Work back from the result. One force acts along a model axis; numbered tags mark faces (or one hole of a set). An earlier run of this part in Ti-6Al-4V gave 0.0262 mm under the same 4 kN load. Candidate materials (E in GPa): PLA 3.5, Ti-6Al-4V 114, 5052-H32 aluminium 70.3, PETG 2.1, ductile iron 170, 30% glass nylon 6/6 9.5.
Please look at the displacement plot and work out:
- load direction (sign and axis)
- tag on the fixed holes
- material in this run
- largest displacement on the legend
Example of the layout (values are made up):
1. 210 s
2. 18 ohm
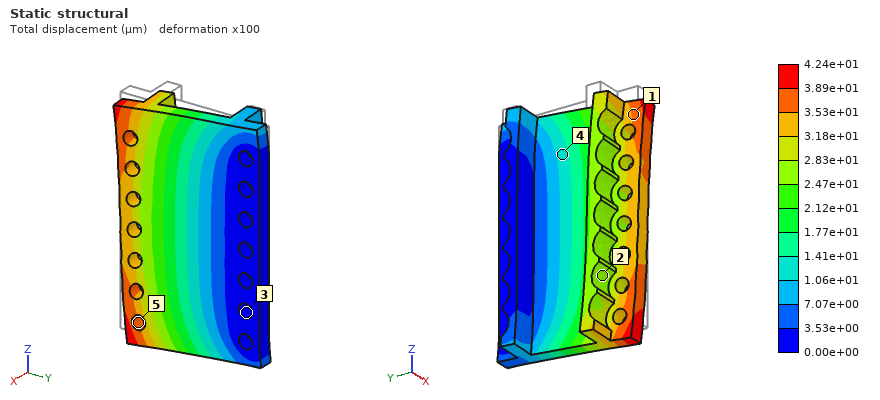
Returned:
1. -Z
2. 3
3. 5052-H32 aluminium
4. 4.24e+01 µm
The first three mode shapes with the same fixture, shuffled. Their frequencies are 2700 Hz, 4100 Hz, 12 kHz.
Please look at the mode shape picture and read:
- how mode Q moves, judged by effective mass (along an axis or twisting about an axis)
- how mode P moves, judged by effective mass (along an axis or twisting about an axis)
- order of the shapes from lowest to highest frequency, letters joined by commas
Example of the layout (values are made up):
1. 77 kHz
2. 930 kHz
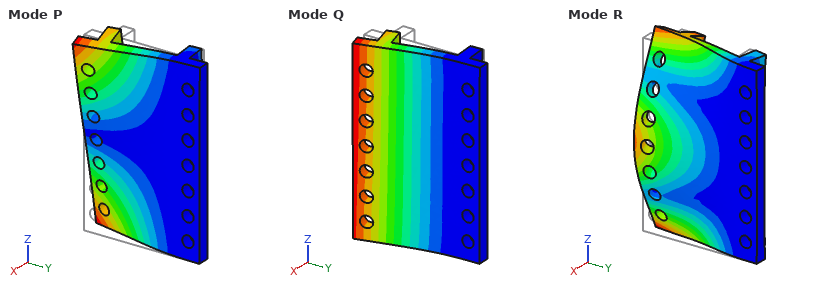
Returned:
1. along X
2. twisting about Y
3. Q, P, R
